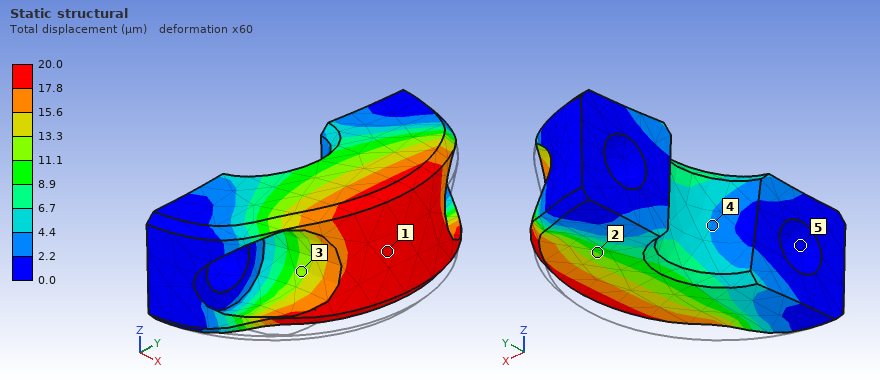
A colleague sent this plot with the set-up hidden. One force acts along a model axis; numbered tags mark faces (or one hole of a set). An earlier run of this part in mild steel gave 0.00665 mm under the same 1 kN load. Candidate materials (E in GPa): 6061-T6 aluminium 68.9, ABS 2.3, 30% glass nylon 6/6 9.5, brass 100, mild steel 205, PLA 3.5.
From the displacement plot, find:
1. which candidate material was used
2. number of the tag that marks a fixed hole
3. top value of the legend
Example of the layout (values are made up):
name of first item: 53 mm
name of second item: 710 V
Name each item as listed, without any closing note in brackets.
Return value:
which candidate material was used: 6061-T6 aluminium
number of the tag that marks a fixed hole: 5
top value of the legend: 20.0 µm
